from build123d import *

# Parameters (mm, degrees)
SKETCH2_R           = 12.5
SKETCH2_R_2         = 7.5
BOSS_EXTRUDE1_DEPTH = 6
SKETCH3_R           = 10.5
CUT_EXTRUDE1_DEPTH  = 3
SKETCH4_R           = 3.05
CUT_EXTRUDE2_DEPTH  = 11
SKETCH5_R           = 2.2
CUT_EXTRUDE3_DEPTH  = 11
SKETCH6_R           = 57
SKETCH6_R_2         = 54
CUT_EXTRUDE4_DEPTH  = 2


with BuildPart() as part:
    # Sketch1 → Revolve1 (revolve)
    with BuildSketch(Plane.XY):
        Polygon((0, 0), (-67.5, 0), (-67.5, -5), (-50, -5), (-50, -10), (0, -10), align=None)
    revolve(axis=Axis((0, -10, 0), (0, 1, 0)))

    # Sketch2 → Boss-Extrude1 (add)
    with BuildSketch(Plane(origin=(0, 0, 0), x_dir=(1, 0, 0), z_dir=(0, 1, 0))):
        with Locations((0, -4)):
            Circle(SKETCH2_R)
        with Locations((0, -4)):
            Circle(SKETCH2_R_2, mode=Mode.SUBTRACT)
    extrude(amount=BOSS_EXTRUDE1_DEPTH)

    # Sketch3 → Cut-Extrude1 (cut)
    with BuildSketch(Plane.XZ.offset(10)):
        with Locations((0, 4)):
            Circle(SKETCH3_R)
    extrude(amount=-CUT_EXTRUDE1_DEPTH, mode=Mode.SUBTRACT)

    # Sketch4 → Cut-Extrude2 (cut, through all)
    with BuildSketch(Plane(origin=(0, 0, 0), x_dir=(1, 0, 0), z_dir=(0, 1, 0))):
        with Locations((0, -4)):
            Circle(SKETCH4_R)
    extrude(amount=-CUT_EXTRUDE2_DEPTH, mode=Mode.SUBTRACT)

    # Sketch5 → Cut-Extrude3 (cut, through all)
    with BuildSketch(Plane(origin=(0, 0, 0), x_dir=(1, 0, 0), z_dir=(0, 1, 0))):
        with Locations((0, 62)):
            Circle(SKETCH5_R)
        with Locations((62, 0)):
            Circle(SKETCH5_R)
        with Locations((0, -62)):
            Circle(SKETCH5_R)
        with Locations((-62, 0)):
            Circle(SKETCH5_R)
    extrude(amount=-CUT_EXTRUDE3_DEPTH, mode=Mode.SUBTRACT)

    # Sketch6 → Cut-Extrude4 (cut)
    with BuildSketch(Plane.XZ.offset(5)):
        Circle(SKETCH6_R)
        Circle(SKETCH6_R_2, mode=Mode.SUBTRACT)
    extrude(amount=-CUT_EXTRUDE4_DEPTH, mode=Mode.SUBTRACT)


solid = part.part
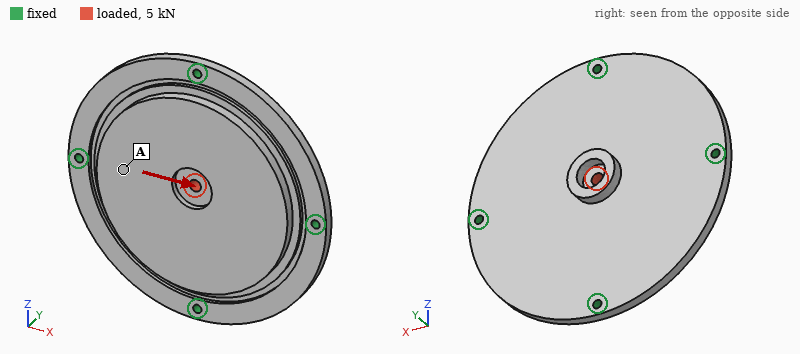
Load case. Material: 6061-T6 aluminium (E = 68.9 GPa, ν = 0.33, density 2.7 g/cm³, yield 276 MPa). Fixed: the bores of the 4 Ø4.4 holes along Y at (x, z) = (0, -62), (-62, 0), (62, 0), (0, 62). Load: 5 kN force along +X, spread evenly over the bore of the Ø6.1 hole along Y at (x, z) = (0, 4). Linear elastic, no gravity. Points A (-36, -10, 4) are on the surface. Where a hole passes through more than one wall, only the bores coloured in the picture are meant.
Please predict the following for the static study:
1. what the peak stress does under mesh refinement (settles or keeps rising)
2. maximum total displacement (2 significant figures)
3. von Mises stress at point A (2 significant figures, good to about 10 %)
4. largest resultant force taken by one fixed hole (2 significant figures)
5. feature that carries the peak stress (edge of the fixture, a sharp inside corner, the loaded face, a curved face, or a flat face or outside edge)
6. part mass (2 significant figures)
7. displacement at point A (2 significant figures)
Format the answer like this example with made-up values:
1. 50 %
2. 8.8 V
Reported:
1. keeps rising
2. 13 µm
3. 5.0 MPa
4. 1.4 kN
5. edge of the fixture
6. 290 g
7. 7.3 µm
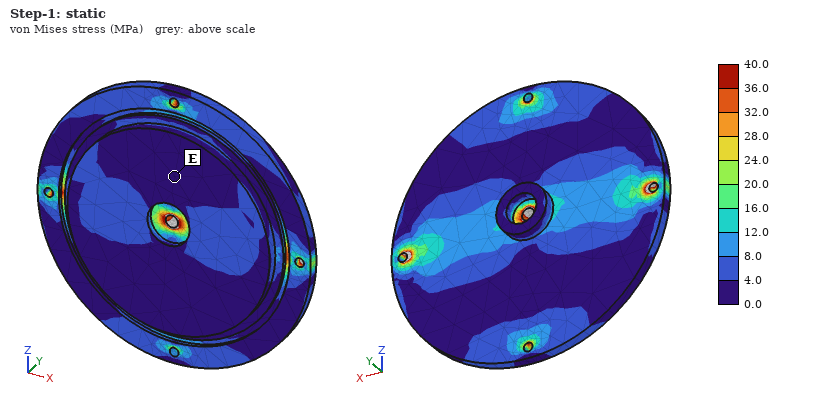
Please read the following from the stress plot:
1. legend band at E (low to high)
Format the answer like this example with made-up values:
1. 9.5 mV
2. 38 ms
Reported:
1. 0.0 to 4.0 MPa
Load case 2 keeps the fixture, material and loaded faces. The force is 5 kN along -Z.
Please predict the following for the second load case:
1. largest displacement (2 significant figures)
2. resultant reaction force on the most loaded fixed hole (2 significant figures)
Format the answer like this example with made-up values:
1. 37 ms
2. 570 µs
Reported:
1. 13 µm
2. 1.5 kN
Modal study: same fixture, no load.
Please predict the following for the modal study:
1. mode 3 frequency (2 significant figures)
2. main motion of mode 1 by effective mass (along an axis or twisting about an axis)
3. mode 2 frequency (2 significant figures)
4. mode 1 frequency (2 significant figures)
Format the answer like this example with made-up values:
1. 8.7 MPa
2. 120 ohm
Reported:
1. 3700 Hz
2. along Y
3. 3700 Hz
4. 2700 Hz
